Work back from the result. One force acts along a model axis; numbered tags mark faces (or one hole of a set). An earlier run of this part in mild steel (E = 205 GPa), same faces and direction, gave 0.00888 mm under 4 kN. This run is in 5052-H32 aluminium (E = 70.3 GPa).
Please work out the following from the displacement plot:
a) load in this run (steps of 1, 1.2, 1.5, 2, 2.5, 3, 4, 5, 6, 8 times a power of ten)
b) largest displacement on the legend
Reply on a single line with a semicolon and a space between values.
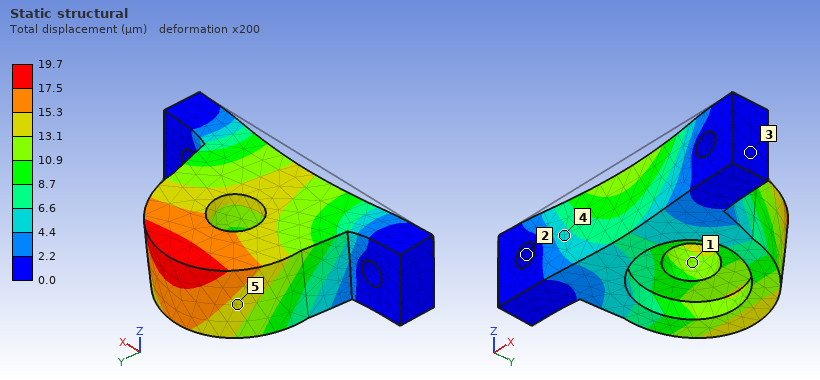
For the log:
3 kN; 19.7 µm
